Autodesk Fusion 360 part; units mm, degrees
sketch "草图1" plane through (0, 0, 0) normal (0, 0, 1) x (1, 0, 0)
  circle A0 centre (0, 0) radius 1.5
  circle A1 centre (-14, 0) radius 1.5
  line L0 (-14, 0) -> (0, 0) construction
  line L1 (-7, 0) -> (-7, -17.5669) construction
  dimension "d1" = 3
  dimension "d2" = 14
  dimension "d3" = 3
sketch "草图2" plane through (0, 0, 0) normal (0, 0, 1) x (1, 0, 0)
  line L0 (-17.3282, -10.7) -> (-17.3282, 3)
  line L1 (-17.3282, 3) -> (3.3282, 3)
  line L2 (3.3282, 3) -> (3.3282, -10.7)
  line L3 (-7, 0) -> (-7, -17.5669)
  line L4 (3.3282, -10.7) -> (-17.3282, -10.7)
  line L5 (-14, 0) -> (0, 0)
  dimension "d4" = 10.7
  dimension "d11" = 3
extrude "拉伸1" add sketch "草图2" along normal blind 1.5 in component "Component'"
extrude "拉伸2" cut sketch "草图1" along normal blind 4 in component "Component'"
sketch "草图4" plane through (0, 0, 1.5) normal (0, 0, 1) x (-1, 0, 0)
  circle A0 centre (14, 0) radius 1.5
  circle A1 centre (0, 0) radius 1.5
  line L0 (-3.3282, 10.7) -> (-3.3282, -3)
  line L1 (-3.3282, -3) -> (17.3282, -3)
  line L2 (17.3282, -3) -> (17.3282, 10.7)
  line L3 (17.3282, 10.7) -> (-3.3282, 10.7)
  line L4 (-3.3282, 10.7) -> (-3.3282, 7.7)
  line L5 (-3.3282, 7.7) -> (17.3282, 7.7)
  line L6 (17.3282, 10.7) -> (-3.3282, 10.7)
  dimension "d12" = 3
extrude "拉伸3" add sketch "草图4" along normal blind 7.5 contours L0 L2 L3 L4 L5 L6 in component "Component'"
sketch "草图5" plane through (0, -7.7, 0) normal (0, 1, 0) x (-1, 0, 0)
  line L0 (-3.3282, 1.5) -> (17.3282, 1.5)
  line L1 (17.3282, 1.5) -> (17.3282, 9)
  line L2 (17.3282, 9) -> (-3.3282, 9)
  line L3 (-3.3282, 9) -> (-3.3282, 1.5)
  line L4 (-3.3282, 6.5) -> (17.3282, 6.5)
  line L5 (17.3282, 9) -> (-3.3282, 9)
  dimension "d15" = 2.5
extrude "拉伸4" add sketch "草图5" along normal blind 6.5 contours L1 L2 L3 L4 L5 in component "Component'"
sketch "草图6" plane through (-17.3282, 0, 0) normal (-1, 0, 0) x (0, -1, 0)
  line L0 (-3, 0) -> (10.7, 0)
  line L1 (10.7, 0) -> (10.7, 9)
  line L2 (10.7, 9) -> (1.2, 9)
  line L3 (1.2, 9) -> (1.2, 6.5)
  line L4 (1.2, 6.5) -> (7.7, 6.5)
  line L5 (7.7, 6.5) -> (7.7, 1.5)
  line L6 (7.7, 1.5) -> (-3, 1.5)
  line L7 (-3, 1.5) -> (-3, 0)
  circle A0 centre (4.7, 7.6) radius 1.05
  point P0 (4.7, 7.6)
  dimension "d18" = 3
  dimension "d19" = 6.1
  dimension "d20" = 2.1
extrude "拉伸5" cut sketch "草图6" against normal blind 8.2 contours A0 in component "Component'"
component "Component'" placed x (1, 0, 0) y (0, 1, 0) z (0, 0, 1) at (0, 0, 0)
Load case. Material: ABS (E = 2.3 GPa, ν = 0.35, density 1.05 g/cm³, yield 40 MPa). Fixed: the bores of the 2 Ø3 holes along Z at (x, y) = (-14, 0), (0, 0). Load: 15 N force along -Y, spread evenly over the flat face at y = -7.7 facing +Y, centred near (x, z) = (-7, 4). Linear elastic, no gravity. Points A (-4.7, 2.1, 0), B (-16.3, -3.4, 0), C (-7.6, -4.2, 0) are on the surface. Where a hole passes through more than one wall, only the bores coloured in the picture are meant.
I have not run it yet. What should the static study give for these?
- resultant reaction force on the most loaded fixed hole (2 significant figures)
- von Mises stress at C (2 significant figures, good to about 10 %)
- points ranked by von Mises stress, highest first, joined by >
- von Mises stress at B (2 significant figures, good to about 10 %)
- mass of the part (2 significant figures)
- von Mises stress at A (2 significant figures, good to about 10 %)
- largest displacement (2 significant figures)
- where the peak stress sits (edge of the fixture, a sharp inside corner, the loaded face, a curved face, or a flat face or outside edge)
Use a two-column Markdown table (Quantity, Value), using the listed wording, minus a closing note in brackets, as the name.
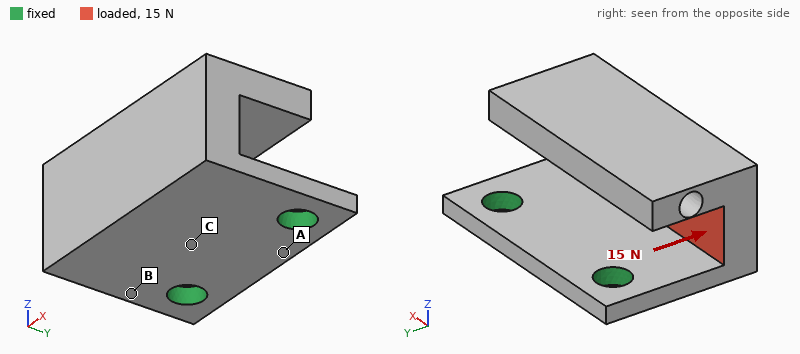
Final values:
| Quantity | Value |
|---|---|
| resultant reaction force on the most loaded fixed hole | 7.7 N |
| von Mises stress at C | 4.6 MPa |
| points ranked by von Mises stress, highest first, joined by > | B > C > A |
| von Mises stress at B | 6.2 MPa |
| mass of the part | 1.2 g |
| von Mises stress at A | 1.2 MPa |
| largest displacement | 0.28 mm |
| where the peak stress sits | a flat face or outside edge |
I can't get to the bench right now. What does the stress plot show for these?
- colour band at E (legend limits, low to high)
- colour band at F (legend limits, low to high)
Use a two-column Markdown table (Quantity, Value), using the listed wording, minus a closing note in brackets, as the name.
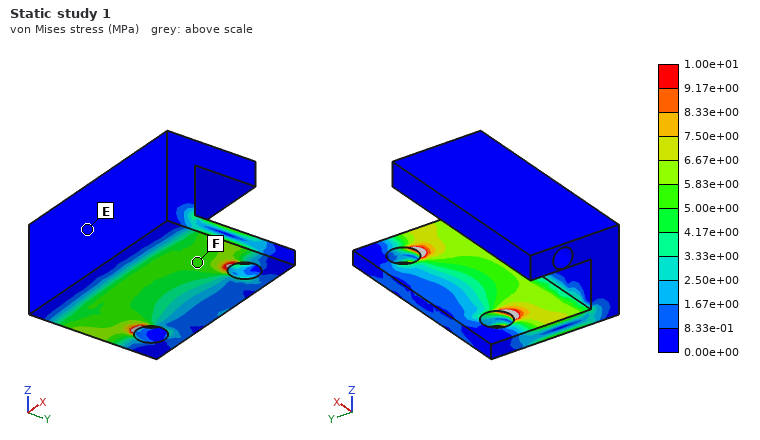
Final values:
| Quantity | Value |
|---|---|
| colour band at E | 0.00e+00 to 8.33e-01 MPa |
| colour band at F | 5.00e+00 to 5.83e+00 MPa |
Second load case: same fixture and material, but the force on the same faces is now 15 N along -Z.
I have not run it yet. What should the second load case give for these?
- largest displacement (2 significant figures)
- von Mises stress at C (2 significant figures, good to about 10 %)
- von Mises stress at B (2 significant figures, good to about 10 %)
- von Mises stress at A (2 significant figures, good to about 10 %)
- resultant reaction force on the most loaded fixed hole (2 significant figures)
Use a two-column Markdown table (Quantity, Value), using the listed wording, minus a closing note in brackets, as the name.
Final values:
| Quantity | Value |
|---|---|
| largest displacement | 0.30 mm |
| von Mises stress at C | 4.6 MPa |
| von Mises stress at B | 9.3 MPa |
| von Mises stress at A | 2.1 MPa |
| resultant reaction force on the most loaded fixed hole | 7.5 N |
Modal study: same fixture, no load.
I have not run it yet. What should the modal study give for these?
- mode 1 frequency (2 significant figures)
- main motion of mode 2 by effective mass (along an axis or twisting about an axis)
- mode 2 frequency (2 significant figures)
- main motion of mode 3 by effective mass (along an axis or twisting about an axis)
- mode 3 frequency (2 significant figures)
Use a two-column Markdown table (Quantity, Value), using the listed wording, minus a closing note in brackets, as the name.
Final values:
| Quantity | Value |
|---|---|
| mode 1 frequency | 1000 Hz |
| main motion of mode 2 by effective mass | along X |
| mode 2 frequency | 2100 Hz |
| main motion of mode 3 by effective mass | along Z |
| mode 3 frequency | 2900 Hz |
